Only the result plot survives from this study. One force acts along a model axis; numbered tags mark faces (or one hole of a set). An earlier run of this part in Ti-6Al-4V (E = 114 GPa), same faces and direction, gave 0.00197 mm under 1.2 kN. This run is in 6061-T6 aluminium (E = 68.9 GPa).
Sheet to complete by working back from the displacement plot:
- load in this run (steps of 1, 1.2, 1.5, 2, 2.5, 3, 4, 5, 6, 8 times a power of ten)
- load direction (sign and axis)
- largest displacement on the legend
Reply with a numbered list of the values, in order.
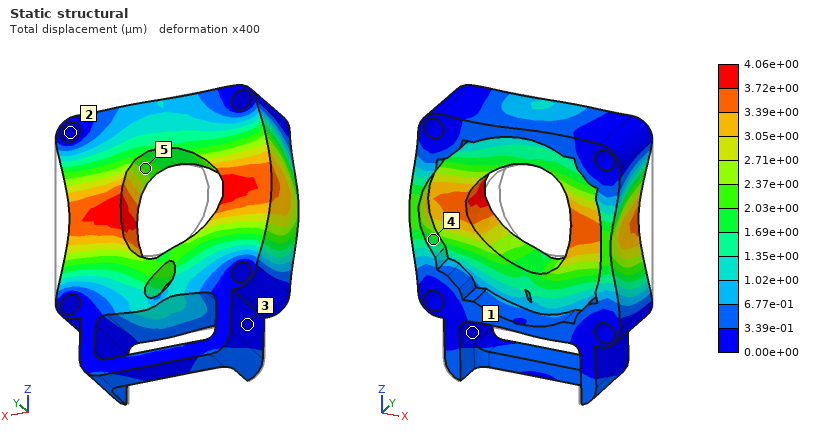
1. 1.5 kN
2. -X
3. 4.06e+00 µm
